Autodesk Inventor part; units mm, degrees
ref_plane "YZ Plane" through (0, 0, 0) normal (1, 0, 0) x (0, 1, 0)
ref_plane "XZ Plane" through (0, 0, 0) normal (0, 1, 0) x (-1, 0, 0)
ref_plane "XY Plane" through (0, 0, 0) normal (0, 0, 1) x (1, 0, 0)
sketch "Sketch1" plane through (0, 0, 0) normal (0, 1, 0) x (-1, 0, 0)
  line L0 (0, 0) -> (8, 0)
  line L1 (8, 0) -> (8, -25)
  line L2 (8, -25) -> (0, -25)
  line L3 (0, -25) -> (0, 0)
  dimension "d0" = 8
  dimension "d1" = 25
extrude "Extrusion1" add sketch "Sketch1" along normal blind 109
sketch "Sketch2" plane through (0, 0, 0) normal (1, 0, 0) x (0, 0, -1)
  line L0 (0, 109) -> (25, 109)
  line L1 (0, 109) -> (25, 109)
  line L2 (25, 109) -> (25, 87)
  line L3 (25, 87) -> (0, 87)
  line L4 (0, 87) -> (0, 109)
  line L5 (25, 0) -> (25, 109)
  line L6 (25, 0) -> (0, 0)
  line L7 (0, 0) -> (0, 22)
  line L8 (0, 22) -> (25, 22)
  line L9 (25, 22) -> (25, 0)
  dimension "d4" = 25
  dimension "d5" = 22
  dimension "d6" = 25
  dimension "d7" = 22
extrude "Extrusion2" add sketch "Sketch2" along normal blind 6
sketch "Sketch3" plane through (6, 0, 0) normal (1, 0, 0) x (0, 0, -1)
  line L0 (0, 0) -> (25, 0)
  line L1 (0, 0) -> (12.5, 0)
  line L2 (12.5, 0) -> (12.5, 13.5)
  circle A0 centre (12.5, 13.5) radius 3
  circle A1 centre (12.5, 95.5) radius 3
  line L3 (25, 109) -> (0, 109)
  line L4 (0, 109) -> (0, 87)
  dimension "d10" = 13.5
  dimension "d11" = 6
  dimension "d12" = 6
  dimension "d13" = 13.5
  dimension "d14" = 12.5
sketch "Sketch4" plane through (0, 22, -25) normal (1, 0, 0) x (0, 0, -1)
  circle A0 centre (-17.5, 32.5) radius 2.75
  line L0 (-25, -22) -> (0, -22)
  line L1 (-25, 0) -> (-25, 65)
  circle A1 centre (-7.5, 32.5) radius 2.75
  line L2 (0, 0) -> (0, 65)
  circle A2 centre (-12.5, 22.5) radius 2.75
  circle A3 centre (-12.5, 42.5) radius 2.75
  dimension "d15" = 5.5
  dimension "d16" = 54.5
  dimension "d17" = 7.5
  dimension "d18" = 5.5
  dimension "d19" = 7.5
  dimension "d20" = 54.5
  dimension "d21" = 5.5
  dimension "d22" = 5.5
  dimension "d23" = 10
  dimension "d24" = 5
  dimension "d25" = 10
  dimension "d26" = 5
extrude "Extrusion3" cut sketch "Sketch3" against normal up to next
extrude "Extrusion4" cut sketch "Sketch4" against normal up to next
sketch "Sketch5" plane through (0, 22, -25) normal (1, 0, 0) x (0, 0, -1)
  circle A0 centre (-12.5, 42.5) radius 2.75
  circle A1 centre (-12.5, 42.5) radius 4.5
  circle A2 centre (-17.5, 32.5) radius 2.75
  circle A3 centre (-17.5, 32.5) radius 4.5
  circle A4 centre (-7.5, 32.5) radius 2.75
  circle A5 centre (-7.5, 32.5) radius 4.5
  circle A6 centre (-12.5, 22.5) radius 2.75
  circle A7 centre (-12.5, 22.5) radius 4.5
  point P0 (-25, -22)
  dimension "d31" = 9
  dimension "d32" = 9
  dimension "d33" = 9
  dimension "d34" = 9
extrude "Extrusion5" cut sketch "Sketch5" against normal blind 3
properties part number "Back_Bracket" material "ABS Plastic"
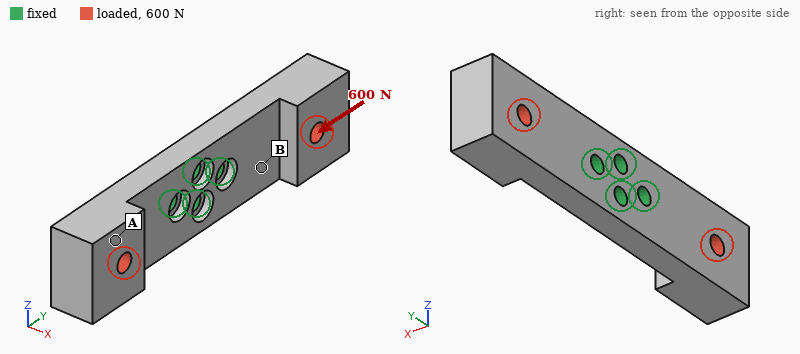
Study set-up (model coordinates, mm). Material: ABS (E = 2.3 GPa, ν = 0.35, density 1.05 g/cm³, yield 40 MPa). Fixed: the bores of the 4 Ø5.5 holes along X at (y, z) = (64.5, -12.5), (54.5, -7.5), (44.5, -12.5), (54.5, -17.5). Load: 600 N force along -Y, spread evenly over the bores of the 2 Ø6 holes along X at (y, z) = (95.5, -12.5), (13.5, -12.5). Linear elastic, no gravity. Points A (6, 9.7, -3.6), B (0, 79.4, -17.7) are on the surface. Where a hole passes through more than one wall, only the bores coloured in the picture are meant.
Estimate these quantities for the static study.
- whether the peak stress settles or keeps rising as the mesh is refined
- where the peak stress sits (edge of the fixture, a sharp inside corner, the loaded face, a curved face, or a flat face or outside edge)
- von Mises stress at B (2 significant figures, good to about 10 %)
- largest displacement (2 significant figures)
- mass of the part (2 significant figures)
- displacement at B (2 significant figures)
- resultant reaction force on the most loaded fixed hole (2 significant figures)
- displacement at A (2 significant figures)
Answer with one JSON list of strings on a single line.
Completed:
["keeps rising", "edge of the fixture", "4.7 MPa", "0.42 mm", "28 g", "0.091 mm", "170 N", "0.32 mm"]
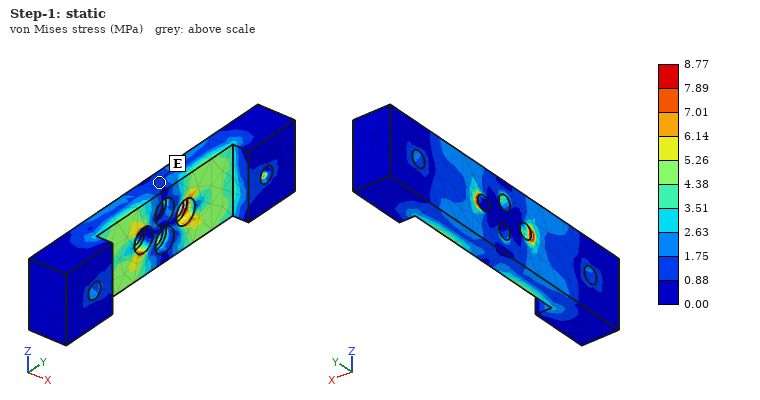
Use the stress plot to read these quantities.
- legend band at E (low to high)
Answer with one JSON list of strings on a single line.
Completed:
["0.88 to 1.75 MPa"]
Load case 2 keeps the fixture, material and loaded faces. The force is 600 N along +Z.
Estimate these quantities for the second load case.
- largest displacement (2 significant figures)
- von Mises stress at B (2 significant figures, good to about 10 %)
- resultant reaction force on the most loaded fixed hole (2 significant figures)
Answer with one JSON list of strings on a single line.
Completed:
["0.51 mm", "6.7 MPa", "430 N"]
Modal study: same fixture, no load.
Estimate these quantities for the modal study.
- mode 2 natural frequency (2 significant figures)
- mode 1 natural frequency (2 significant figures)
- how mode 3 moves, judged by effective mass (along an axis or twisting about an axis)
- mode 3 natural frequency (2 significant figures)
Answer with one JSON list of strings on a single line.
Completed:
["650 Hz", "650 Hz", "twisting about X", "1400 Hz"]
